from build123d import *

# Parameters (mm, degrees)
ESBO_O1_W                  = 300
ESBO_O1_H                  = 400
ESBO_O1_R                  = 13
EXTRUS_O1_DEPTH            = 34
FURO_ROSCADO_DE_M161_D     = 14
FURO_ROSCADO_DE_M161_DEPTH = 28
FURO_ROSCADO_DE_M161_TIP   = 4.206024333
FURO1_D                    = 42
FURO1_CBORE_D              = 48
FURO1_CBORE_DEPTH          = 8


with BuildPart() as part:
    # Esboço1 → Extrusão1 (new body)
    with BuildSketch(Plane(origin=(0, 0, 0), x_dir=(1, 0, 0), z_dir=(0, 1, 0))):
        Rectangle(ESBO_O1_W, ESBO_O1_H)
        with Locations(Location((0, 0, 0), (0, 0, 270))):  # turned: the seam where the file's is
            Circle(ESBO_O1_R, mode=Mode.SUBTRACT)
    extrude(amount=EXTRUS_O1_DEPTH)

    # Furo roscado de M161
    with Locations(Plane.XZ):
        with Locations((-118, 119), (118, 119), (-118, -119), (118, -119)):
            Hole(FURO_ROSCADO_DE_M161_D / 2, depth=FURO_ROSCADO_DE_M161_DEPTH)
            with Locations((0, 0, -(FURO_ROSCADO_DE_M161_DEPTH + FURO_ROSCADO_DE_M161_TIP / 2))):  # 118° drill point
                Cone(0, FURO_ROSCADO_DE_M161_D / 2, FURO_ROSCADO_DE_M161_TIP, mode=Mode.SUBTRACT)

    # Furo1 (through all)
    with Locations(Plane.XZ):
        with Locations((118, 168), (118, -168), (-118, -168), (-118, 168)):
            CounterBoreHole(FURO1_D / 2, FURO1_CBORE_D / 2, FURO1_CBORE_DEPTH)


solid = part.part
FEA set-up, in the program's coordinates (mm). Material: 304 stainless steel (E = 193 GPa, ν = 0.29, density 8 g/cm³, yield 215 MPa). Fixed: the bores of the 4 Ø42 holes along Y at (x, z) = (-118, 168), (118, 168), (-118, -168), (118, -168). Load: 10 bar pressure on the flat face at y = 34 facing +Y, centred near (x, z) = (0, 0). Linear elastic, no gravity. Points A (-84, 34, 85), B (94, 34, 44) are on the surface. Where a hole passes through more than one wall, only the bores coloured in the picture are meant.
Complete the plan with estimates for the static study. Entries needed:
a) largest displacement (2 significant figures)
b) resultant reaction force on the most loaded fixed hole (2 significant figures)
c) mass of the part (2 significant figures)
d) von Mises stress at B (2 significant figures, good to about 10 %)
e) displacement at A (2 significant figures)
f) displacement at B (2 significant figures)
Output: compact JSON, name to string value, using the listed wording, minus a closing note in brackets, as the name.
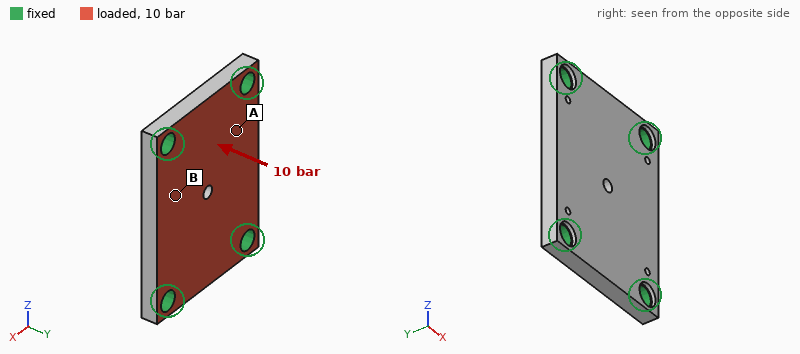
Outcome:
{"largest displacement": "81 µm", "resultant reaction force on the most loaded fixed hole": "29 kN", "mass of the part": "31 kg", "von Mises stress at B": "20 MPa", "displacement at A": "45 µm", "displacement at B": "62 µm"}
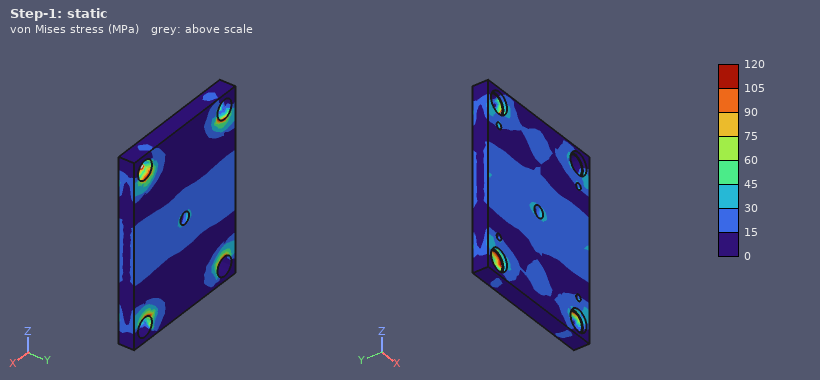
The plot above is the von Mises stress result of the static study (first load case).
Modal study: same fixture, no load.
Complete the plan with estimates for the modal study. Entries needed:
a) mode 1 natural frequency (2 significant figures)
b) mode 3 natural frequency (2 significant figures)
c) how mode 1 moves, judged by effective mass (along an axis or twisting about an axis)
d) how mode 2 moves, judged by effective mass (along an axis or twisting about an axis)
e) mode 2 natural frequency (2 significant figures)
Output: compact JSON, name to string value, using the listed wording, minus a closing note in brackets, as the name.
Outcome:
{"mode 1 natural frequency": "1300 Hz", "mode 3 natural frequency": "2700 Hz", "how mode 1 moves, judged by effective mass": "along Y", "how mode 2 moves, judged by effective mass": "twisting about Z", "mode 2 natural frequency": "1800 Hz"}
